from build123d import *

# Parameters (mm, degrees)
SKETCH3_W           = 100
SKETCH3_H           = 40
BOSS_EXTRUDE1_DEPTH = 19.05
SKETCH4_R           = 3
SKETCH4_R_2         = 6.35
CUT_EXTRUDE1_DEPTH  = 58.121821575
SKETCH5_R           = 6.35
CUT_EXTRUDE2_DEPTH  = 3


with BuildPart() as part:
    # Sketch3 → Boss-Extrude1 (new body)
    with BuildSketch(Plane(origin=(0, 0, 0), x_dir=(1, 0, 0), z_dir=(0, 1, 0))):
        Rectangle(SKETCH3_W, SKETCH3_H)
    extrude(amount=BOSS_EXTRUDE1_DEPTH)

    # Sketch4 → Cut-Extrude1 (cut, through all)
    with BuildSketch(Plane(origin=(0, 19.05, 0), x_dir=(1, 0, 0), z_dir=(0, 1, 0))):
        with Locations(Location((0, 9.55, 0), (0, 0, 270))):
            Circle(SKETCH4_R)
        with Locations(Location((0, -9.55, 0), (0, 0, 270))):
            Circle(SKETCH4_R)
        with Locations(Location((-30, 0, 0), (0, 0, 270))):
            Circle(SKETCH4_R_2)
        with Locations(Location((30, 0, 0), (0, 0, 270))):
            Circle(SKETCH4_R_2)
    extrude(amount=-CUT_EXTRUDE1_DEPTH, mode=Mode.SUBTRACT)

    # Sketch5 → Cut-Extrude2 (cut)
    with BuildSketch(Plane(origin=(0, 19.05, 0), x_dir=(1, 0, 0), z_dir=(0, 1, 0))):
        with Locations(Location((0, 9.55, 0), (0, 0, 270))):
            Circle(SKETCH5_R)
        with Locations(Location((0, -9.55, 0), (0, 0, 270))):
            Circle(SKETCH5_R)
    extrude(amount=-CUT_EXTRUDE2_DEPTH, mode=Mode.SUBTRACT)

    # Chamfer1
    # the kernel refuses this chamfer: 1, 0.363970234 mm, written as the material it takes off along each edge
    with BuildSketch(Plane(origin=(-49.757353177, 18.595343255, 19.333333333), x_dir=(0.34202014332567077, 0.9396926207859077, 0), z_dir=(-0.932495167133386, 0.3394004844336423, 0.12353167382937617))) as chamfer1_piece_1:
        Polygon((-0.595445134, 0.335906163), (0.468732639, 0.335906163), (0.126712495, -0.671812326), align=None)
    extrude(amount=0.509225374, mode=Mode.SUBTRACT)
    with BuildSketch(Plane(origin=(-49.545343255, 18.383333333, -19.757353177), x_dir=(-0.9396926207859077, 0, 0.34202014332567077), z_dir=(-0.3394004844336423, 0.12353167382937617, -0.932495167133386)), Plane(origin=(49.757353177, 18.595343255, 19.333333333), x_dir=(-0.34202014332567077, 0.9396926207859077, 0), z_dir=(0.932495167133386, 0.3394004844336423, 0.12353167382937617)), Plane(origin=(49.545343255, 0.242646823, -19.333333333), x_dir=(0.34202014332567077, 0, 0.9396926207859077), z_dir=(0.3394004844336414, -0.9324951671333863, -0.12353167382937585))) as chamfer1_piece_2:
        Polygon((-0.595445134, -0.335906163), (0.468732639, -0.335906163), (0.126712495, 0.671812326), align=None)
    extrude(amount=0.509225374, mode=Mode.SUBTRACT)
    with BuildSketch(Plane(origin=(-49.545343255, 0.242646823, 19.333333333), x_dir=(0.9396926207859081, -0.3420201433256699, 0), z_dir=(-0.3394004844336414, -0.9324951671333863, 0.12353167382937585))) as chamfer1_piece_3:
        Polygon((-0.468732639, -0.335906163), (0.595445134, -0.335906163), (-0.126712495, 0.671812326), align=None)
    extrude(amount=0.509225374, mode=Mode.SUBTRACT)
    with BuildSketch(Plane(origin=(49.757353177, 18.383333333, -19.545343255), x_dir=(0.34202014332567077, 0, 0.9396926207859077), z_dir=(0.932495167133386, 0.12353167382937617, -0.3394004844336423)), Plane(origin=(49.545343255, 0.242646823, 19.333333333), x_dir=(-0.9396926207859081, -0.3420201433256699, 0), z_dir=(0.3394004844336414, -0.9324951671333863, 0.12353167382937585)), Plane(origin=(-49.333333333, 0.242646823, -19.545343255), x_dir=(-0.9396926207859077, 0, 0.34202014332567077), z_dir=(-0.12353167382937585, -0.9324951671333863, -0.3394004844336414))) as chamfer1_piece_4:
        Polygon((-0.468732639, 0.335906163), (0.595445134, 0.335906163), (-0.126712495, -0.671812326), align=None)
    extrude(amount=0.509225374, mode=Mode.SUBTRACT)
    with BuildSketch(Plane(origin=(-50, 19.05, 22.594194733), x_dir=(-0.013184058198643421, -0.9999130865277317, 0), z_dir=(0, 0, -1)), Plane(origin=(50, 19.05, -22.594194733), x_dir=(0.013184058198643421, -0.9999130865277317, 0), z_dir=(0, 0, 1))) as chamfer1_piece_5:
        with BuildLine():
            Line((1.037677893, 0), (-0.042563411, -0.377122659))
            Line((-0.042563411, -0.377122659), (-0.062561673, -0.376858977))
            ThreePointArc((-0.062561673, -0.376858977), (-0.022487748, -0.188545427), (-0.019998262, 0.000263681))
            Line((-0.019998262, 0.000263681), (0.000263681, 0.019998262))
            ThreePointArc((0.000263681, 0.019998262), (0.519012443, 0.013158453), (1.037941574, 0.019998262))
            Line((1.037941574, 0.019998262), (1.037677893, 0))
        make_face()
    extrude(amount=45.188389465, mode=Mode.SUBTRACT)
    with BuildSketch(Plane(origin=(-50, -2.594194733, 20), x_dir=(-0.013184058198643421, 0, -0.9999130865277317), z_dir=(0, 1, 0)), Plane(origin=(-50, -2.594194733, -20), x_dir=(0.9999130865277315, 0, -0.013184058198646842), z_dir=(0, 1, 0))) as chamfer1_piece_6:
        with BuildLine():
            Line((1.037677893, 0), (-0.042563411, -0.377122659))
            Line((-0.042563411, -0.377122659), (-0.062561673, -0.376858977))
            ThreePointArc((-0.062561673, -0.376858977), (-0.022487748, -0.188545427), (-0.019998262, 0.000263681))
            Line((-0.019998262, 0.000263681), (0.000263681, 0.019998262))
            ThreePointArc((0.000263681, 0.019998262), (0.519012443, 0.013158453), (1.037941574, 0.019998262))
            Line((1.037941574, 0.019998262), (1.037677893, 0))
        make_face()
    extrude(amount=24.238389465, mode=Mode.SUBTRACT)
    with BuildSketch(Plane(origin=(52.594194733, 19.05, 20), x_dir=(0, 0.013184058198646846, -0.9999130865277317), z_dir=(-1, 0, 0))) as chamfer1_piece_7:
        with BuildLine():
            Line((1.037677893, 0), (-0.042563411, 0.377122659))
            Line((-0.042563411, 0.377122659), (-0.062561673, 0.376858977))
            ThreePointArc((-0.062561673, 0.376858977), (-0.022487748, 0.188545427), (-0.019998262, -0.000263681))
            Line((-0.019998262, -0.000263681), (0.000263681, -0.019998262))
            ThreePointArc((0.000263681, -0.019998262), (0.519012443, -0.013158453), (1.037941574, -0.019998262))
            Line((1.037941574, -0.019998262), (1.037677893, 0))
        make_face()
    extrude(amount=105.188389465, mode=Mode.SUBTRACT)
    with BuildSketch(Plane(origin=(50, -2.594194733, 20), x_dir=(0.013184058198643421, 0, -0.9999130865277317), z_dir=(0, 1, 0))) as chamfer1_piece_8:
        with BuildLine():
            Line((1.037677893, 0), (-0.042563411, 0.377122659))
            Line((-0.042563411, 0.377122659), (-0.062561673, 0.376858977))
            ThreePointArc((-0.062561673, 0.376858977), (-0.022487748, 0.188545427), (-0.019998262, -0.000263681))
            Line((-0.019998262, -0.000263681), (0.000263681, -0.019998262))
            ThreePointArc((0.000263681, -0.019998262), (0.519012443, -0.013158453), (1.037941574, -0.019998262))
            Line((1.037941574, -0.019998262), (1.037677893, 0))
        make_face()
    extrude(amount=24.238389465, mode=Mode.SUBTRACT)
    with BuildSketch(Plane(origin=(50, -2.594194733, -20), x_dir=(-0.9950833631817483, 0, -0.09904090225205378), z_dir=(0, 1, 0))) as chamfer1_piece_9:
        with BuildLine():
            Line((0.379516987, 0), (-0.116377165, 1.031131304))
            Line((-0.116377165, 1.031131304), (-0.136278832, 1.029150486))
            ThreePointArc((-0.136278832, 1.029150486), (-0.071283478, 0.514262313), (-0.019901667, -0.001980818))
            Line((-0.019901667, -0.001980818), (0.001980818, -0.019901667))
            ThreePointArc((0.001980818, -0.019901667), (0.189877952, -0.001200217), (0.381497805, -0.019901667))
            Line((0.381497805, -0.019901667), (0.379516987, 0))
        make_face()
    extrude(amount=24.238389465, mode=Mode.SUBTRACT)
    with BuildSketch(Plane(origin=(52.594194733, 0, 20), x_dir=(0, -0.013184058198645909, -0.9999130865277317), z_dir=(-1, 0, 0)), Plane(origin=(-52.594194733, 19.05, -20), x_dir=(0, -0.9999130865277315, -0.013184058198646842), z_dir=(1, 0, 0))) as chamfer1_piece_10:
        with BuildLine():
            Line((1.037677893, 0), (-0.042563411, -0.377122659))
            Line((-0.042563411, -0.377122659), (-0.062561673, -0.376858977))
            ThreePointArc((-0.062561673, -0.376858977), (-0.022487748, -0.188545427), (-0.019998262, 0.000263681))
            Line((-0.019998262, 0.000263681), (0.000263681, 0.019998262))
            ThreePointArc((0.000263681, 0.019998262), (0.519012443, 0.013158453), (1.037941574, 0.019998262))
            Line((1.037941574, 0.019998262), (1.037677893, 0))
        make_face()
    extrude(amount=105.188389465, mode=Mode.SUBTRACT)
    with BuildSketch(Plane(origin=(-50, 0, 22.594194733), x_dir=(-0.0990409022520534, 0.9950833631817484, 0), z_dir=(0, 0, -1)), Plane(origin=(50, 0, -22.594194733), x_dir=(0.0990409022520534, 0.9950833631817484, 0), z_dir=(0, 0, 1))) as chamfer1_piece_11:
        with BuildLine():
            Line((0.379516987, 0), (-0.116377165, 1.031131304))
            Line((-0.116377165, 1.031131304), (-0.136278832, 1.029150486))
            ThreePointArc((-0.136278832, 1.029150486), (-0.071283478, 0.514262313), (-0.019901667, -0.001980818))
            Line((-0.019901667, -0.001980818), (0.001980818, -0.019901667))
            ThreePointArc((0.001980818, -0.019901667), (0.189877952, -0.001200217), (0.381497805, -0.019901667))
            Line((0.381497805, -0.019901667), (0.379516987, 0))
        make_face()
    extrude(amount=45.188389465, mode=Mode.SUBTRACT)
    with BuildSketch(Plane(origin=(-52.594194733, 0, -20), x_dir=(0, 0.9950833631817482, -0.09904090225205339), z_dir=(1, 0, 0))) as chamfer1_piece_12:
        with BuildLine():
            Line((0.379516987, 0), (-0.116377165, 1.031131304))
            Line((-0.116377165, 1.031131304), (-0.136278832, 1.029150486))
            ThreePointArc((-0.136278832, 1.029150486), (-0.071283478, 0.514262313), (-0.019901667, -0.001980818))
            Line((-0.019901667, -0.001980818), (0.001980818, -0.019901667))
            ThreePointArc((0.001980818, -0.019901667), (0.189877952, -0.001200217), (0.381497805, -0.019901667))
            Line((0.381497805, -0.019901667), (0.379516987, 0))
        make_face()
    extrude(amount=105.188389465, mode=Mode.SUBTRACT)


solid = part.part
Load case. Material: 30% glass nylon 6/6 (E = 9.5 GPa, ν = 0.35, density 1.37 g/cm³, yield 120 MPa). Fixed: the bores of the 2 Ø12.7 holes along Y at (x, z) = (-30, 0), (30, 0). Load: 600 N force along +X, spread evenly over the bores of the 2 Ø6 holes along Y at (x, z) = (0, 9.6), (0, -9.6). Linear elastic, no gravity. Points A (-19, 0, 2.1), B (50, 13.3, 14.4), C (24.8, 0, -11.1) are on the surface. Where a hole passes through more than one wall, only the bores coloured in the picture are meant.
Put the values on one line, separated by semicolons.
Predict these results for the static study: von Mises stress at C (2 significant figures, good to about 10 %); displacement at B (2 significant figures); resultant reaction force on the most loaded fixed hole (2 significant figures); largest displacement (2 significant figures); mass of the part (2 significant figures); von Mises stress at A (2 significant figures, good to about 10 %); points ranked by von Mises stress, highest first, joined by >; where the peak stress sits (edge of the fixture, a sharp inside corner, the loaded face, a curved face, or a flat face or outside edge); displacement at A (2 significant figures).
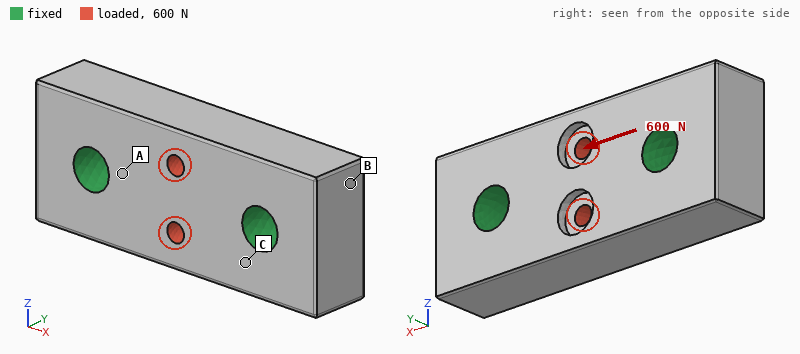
0.28 MPa; 0.37 µm; 300 N; 1.8 µm; 95 g; 0.67 MPa; A > C > B; the loaded face; 0.41 µm
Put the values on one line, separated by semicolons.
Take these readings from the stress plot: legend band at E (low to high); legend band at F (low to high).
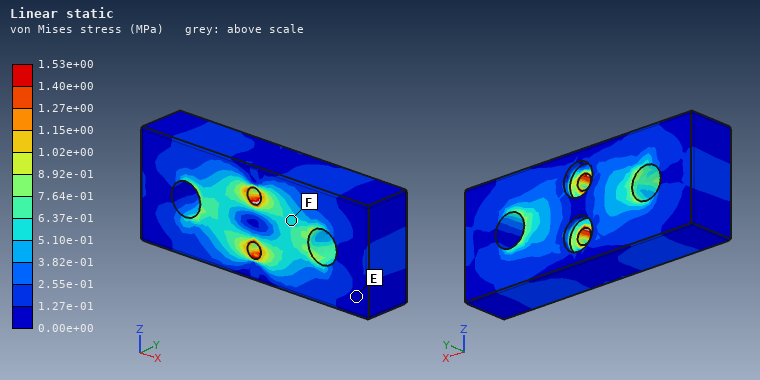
0.00e+00 to 1.27e-01 MPa; 5.10e-01 to 6.37e-01 MPa
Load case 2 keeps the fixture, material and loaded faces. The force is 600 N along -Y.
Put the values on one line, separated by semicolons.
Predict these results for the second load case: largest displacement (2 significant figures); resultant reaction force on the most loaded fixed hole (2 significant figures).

7.5 µm; 300 N
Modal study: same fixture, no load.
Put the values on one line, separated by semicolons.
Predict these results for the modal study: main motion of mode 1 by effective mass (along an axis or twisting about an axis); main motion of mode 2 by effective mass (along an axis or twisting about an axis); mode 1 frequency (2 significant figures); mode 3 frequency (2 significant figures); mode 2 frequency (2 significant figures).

along Y; twisting about X; 9900 Hz; 11 kHz; 10 kHz
